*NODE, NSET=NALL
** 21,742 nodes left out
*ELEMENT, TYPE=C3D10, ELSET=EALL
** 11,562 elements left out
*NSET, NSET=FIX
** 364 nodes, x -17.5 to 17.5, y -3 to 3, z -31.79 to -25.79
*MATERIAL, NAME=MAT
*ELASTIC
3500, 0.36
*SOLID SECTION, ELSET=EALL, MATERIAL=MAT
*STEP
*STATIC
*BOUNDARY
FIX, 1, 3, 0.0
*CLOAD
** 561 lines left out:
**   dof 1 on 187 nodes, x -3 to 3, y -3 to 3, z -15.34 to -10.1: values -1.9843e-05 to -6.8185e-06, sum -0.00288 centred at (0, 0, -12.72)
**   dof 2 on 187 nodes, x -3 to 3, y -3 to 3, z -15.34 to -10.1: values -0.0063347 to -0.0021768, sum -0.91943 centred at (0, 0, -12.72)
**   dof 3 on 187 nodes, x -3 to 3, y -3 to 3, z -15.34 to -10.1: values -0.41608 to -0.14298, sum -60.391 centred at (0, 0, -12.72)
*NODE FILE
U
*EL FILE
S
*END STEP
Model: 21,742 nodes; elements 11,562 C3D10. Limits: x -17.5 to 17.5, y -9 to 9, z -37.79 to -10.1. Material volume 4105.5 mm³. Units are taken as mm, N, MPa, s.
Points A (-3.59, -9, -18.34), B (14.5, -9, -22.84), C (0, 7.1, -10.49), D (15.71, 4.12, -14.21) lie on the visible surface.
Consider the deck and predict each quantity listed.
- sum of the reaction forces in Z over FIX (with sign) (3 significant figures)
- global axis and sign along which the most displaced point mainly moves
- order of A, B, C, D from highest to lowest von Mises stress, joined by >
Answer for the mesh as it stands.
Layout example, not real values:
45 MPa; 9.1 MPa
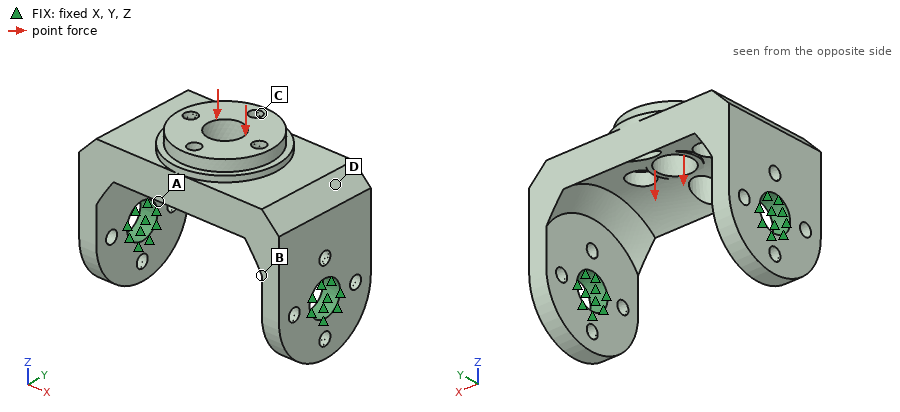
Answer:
60.4 N; -Z; C > A > B > D
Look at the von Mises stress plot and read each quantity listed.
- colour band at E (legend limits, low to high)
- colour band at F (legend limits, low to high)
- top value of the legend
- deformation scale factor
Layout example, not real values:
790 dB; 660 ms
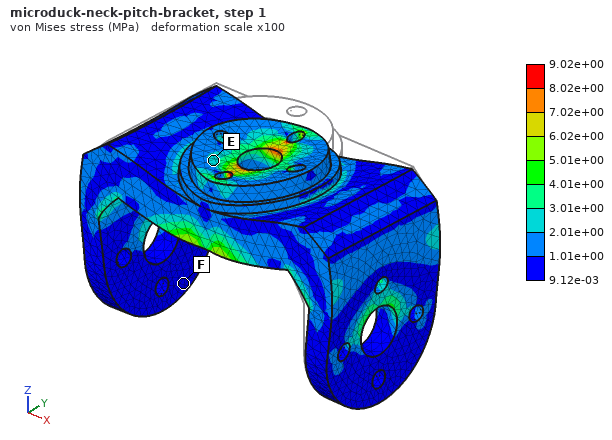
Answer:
2.01e+00 to 3.01e+00 MPa; 9.12e-03 to 1.01e+00 MPa; 9.02e+00 MPa; 100
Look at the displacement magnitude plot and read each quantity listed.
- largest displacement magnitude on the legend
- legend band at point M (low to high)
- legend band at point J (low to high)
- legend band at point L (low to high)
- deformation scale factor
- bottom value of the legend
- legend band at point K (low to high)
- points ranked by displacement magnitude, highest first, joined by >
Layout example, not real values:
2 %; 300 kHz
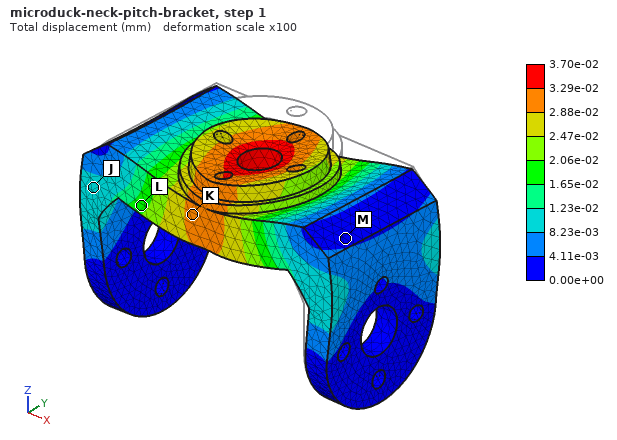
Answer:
3.70e-02 mm; 0.00e+00 to 4.11e-03 mm; 8.23e-03 to 1.23e-02 mm; 1.65e-02 to 2.06e-02 mm; 100; 0.00e+00 mm; 2.88e-02 to 3.29e-02 mm; K > L > J > M
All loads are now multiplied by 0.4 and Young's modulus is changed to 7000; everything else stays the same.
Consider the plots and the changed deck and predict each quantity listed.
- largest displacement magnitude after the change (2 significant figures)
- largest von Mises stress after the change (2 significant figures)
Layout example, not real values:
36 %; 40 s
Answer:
0.0074 mm; 3.6 MPa
